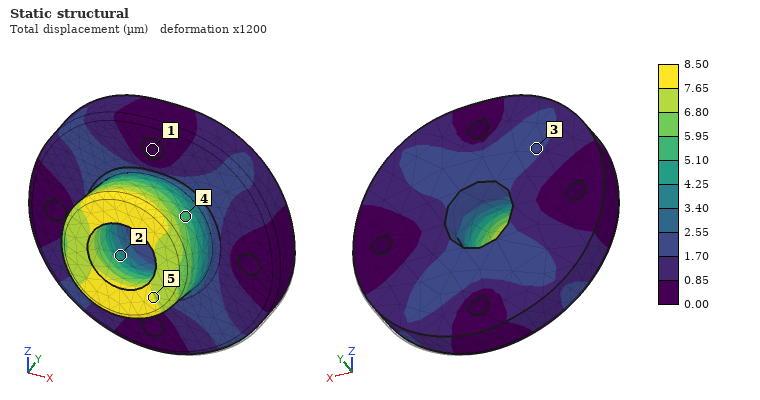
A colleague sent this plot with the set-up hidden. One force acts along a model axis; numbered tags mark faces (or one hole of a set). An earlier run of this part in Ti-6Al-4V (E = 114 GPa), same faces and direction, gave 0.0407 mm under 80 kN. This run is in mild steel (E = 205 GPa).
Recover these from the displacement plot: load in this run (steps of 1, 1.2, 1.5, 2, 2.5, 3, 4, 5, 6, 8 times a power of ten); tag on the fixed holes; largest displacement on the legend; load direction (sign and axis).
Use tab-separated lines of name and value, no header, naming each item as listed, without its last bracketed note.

load in this run	30 kN
tag on the fixed holes	1
largest displacement on the legend	8.50 µm
load direction	+Z
